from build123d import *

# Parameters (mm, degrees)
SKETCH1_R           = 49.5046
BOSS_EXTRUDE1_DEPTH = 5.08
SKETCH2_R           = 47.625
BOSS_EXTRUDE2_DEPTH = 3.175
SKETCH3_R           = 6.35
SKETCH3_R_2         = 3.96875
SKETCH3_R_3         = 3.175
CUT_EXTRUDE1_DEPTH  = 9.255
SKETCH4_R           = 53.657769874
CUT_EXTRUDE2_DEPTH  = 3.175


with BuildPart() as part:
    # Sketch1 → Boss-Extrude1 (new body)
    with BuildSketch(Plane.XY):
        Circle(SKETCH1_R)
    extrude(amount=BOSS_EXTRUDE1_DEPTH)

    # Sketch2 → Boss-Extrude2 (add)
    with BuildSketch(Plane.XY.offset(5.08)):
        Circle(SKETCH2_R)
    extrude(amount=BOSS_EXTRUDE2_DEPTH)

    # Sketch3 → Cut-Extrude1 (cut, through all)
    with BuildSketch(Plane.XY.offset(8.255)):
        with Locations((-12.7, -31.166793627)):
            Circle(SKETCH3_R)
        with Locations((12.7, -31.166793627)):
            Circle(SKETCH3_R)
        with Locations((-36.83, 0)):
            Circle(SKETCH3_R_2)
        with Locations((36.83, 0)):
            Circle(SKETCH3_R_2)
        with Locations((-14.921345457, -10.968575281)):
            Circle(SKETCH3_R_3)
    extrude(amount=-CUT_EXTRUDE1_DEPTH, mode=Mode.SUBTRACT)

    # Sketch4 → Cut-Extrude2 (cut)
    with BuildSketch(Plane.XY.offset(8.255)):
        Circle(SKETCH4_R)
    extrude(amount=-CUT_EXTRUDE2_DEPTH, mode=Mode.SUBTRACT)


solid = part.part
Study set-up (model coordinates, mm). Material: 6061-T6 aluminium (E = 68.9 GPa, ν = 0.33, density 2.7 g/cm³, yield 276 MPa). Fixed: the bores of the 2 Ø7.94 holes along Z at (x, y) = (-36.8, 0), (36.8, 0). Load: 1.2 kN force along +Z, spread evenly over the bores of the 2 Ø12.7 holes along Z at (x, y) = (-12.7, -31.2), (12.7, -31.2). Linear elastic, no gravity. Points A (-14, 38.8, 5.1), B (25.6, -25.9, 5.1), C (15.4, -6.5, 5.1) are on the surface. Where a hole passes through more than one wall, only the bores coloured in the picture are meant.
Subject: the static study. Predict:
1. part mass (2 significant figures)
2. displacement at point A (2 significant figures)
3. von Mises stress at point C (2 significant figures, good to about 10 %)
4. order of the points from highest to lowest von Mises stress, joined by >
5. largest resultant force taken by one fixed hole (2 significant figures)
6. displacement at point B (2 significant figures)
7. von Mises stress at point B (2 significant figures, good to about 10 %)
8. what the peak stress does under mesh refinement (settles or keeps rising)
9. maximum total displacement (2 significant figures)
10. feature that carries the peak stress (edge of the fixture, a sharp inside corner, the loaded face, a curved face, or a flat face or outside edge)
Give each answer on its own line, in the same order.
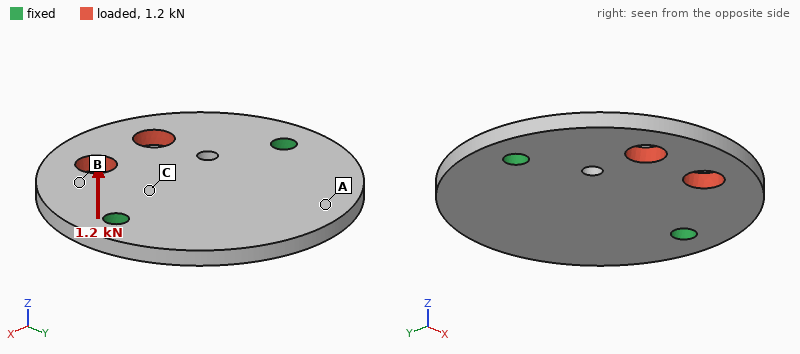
100 g
0.090 mm
55 MPa
C > B > A
600 N
0.19 mm
33 MPa
keeps rising
0.54 mm
edge of the fixture
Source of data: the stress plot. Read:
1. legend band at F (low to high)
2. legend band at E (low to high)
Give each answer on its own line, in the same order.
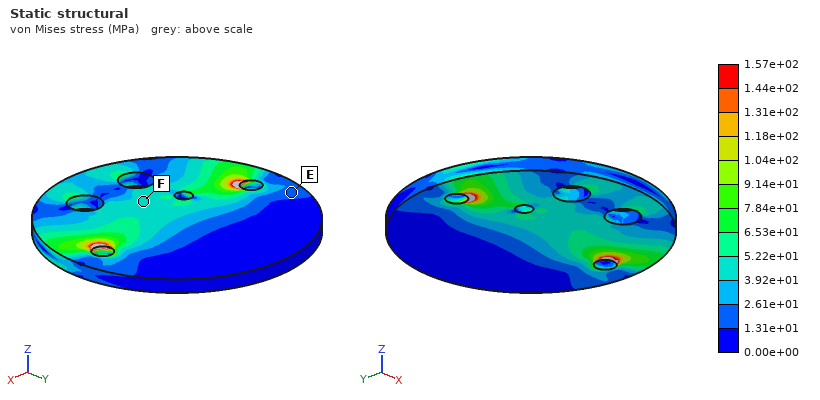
3.92e+01 to 5.22e+01 MPa
1.31e+01 to 2.61e+01 MPa
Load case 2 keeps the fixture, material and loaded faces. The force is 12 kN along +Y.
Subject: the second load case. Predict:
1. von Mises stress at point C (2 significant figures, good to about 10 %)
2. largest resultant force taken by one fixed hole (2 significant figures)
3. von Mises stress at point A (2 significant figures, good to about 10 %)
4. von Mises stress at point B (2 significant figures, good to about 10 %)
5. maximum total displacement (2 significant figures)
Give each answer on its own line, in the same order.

28 MPa
6.1 kN
11 MPa
37 MPa
38 µm
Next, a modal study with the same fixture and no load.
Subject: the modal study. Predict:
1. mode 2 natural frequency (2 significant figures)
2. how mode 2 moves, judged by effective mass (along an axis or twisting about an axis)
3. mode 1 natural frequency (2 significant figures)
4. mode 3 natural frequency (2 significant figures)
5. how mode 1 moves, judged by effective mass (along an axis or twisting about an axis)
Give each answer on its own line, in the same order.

2200 Hz
along Z
1700 Hz
4500 Hz
twisting about X
